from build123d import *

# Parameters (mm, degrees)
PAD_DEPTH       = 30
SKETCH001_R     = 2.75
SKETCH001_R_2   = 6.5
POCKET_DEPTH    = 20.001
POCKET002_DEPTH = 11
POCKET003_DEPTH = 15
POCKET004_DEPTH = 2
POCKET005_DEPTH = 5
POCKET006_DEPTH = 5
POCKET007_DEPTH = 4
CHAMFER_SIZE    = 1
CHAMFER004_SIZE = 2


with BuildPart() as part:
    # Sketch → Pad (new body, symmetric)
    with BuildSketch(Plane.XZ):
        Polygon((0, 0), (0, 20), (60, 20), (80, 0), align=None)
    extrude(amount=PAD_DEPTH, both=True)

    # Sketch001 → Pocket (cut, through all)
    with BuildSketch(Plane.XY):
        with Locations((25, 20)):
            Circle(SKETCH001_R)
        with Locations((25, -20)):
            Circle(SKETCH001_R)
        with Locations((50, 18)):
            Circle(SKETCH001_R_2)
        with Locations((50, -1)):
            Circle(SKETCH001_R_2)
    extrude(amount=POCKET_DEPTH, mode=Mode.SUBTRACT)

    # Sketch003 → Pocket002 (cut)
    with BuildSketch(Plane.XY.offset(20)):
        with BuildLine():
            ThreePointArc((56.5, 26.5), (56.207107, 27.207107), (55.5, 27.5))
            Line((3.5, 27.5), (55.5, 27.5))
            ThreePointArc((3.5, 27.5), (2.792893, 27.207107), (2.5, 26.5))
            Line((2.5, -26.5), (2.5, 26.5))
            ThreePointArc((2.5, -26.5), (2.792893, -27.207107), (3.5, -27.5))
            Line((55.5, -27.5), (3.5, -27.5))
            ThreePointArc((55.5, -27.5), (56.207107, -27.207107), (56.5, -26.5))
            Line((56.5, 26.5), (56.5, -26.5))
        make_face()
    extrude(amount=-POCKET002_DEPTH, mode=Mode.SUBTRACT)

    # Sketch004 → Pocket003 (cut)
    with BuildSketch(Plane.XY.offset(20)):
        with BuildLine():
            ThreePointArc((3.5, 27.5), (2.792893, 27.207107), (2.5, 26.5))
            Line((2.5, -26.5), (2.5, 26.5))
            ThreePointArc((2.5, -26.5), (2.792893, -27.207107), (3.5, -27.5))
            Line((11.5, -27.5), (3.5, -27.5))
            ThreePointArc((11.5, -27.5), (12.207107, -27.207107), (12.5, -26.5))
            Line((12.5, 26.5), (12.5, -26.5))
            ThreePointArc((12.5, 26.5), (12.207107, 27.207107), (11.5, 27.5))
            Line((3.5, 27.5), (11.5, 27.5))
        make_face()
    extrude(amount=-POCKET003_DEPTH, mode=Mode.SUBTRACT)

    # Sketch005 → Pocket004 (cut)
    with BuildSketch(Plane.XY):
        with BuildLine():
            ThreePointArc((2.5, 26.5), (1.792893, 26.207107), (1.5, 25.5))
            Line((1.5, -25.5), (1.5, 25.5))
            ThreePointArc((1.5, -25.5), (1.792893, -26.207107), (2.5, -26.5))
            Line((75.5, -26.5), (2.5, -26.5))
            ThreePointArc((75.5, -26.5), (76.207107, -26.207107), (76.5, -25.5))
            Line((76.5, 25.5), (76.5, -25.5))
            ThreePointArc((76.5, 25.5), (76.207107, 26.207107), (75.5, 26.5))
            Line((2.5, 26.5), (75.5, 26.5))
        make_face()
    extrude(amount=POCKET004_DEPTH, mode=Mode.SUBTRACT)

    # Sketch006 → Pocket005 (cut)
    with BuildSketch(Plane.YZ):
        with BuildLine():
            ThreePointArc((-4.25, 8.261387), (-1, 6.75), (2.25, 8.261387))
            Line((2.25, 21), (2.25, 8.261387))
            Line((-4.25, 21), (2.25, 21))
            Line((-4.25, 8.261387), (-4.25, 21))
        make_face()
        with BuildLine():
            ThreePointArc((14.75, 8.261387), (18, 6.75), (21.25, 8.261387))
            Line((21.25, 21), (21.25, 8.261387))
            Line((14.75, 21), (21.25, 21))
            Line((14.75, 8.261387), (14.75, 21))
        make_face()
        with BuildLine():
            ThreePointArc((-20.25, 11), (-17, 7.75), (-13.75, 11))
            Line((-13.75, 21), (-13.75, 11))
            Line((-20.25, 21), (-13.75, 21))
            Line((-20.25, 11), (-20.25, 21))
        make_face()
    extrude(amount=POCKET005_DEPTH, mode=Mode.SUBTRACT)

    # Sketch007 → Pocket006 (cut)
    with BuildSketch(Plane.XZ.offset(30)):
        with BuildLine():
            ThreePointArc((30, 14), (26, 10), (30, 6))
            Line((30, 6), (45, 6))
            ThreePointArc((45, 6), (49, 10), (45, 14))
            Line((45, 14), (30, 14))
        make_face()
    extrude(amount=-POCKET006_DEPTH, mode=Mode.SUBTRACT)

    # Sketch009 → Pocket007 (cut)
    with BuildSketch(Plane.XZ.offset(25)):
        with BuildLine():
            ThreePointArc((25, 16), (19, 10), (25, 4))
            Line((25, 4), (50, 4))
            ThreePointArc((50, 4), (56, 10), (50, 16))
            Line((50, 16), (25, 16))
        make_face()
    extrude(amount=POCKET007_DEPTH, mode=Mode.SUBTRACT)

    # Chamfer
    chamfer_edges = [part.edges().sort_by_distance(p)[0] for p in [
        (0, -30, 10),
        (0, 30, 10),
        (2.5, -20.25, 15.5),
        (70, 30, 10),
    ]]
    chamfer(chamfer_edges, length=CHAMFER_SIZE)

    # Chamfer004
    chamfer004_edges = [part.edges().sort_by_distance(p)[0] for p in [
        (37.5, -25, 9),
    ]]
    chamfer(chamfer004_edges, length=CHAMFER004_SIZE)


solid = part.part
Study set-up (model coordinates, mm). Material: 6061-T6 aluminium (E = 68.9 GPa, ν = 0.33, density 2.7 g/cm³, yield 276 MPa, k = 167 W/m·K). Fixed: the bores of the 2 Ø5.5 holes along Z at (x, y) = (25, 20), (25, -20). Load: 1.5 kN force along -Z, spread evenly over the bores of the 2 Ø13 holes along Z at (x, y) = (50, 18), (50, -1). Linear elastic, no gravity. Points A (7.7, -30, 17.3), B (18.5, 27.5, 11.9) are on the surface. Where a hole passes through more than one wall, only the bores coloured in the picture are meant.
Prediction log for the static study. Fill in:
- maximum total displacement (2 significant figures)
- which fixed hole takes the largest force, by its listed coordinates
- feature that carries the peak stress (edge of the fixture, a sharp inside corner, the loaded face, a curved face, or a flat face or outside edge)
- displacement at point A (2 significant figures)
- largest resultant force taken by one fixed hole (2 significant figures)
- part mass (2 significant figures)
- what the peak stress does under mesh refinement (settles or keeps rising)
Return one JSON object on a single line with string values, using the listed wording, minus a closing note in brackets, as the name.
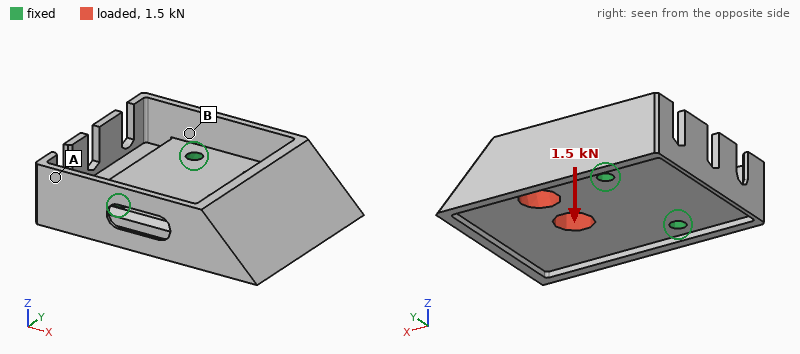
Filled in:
{"maximum total displacement": "0.15 mm", "which fixed hole takes the largest force, by its listed coordinates": "(25, 20)", "feature that carries the peak stress": "edge of the fixture", "displacement at point A": "0.026 mm", "largest resultant force taken by one fixed hole": "1.0 kN", "part mass": "100 g", "what the peak stress does under mesh refinement": "keeps rising"}
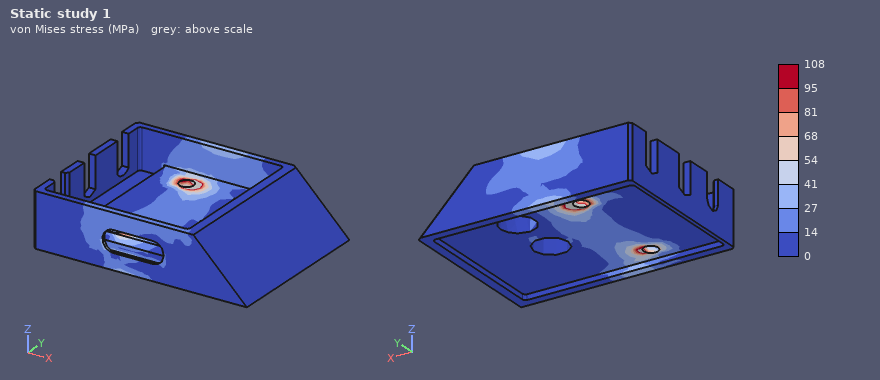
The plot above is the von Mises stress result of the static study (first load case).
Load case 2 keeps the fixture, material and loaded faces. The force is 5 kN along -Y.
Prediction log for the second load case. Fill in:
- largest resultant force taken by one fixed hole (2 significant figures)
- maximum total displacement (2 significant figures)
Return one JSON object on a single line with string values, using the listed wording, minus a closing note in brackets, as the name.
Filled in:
{"largest resultant force taken by one fixed hole": "4.0 kN", "maximum total displacement": "37 µm"}
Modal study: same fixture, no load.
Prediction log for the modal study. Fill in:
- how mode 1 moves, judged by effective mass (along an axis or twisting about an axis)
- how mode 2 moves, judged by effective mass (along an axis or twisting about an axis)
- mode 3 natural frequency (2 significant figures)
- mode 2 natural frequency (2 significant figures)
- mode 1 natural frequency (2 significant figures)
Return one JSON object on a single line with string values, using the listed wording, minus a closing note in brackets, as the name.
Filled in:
{"how mode 1 moves, judged by effective mass": "along Z", "how mode 2 moves, judged by effective mass": "twisting about X", "mode 3 natural frequency": "5800 Hz", "mode 2 natural frequency": "4100 Hz", "mode 1 natural frequency": "2100 Hz"}
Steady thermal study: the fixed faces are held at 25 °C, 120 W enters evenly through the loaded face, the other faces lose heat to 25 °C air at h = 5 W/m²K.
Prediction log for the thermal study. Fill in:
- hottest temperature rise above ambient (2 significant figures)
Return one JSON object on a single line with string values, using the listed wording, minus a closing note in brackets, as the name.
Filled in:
{"hottest temperature rise above ambient": "61 K"}
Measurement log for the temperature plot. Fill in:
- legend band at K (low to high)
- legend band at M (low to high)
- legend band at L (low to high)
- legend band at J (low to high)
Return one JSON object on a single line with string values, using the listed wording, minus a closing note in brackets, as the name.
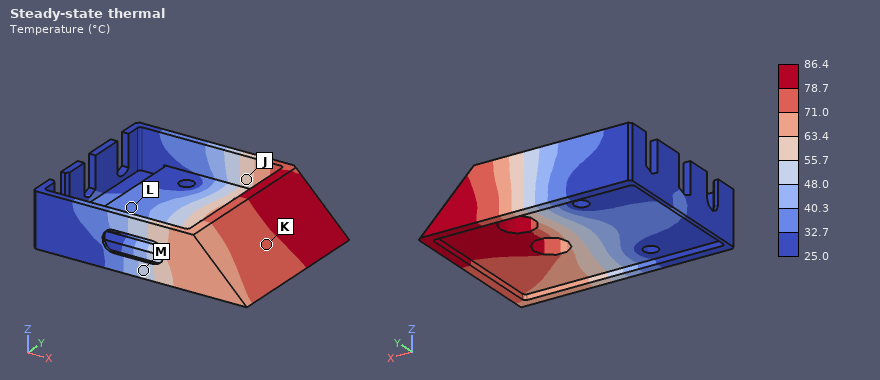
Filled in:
{"legend band at K": "71.0 to 78.7 °C", "legend band at M": "48.0 to 55.7 °C", "legend band at L": "32.7 to 40.3 °C", "legend band at J": "55.7 to 63.4 °C"}
